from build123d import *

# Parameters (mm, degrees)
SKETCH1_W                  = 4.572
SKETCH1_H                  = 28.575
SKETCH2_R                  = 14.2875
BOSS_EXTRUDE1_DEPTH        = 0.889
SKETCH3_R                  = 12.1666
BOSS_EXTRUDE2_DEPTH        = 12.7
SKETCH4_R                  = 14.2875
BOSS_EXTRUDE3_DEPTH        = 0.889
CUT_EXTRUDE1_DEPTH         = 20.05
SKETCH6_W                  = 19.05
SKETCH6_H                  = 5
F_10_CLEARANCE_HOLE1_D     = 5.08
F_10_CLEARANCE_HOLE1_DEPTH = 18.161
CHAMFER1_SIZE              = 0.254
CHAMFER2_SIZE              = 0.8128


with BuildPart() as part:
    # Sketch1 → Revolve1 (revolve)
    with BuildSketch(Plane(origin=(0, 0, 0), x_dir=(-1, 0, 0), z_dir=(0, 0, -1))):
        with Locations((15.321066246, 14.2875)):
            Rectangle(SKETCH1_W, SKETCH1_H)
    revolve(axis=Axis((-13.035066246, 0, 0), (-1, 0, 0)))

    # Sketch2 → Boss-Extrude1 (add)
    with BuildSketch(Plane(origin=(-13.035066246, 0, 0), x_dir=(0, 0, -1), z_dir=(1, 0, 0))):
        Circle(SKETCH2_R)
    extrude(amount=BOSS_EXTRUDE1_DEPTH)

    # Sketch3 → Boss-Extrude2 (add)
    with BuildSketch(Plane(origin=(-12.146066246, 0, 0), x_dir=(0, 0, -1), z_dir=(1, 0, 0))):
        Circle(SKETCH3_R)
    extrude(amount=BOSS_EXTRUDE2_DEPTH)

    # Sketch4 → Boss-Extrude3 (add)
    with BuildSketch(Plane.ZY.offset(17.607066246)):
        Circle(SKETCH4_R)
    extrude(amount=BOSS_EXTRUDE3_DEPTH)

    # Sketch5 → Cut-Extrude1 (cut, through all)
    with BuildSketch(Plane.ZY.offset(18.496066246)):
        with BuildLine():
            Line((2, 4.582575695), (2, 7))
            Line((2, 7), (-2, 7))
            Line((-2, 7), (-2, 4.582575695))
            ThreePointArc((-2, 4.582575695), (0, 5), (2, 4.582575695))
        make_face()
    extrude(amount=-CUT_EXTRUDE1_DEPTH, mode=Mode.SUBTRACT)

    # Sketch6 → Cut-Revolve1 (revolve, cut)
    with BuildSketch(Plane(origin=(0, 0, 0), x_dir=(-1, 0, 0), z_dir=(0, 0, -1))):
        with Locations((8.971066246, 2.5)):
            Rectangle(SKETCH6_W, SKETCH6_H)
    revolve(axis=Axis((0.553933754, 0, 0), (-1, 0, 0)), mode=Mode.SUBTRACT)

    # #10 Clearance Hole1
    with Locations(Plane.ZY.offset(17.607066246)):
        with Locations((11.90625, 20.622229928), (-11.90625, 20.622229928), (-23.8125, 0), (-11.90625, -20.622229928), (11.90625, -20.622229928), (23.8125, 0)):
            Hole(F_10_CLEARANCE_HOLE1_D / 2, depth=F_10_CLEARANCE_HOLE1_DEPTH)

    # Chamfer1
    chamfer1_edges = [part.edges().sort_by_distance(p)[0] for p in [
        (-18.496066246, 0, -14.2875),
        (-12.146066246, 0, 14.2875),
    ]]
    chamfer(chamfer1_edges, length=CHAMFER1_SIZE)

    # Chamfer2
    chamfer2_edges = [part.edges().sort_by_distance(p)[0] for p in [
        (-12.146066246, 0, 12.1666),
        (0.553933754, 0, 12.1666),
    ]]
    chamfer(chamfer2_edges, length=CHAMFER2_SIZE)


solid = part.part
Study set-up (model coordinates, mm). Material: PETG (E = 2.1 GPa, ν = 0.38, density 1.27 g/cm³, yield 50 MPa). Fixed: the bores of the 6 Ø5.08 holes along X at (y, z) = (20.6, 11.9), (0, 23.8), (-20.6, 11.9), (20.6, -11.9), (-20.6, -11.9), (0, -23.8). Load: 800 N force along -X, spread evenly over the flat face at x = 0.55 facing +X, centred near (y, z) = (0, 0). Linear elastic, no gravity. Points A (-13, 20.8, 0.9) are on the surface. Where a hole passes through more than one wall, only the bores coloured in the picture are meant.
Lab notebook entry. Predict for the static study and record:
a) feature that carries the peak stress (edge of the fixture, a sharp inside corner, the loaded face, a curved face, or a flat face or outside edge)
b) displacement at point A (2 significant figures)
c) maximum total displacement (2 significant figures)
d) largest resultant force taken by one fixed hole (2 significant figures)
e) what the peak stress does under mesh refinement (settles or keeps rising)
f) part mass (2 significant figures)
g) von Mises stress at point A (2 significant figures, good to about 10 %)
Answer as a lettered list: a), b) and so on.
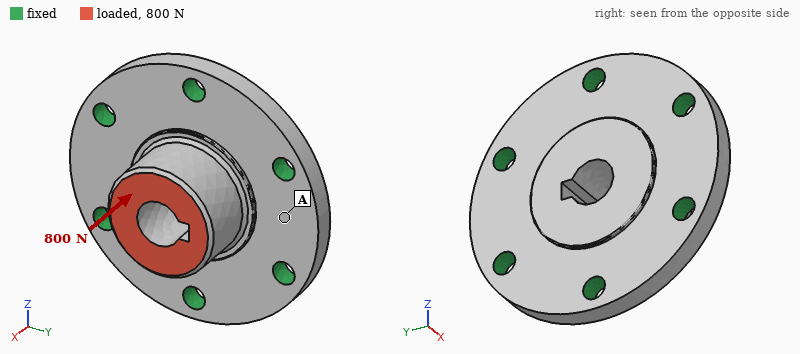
a) edge of the fixture
b) 0.027 mm
c) 0.11 mm
d) 150 N
e) keeps rising
f) 21 g
g) 2.6 MPa
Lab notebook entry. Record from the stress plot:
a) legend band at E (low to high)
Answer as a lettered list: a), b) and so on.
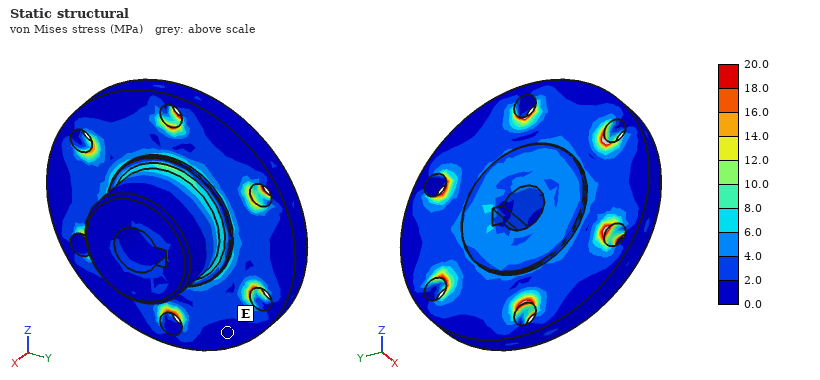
a) 0.0 to 2.0 MPa
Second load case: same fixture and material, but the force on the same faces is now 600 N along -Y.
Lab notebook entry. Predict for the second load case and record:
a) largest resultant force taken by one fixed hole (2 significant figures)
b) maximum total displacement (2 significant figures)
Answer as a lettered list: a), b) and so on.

a) 200 N
b) 0.18 mm
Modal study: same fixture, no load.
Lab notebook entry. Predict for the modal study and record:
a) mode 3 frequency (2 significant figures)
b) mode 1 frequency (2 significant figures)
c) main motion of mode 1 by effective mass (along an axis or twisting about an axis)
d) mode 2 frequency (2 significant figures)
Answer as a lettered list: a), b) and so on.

a) 5200 Hz
b) 4300 Hz
c) along X
d) 5200 Hz
